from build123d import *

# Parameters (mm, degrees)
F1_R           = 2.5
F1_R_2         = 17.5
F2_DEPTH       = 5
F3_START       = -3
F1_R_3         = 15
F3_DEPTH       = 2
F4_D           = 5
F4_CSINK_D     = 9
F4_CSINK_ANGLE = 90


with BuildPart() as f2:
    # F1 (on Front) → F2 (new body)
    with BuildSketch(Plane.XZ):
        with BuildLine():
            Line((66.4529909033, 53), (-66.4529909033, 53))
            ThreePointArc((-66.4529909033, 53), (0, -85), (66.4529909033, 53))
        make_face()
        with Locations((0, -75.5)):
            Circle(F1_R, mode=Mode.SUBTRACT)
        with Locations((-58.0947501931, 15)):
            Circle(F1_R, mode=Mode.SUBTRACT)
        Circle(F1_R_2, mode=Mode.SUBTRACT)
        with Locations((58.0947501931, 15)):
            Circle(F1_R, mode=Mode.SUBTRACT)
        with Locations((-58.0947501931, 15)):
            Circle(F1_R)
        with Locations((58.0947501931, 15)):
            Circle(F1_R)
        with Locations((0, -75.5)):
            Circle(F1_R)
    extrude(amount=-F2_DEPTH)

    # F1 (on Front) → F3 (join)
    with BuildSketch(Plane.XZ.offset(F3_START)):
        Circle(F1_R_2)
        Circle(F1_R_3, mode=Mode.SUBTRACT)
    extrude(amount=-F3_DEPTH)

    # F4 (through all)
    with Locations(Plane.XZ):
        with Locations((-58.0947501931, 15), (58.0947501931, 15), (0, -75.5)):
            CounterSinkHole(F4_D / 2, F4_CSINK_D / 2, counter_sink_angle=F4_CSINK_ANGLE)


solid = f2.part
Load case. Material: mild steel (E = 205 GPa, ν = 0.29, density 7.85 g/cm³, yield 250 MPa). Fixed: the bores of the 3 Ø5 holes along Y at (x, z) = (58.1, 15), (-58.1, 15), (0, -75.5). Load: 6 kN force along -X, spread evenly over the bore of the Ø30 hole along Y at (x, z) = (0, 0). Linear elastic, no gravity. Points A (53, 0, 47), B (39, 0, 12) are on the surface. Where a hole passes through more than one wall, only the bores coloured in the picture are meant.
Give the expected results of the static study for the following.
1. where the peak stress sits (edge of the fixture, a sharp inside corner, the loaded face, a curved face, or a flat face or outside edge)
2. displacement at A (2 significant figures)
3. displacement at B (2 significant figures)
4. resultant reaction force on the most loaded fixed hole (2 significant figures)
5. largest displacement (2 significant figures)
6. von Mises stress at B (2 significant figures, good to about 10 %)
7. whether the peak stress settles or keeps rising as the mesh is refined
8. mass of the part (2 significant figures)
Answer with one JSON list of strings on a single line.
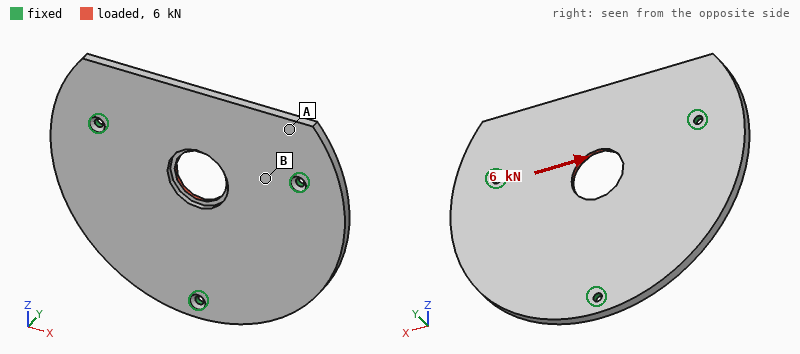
["edge of the fixture", "2.4 µm", "3.6 µm", "2.4 kN", "5.4 µm", "11 MPa", "keeps rising", "740 g"]
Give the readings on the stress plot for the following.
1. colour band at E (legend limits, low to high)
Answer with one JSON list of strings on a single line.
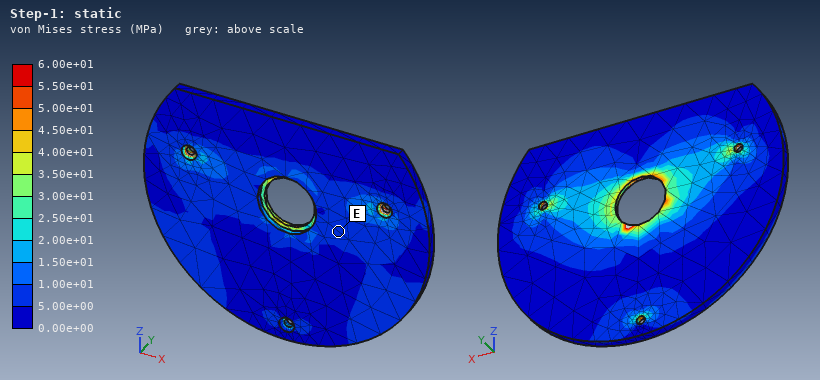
["5.00e+00 to 1.00e+01 MPa"]
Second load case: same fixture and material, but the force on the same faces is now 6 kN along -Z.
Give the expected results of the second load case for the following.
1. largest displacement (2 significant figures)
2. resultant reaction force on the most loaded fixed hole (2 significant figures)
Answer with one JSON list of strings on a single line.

["18 µm", "2.1 kN"]
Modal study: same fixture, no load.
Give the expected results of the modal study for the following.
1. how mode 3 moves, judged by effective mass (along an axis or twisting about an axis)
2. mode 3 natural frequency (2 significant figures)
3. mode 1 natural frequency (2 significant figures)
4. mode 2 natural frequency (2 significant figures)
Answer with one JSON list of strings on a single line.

["along Y", "1500 Hz", "1200 Hz", "1300 Hz"]
